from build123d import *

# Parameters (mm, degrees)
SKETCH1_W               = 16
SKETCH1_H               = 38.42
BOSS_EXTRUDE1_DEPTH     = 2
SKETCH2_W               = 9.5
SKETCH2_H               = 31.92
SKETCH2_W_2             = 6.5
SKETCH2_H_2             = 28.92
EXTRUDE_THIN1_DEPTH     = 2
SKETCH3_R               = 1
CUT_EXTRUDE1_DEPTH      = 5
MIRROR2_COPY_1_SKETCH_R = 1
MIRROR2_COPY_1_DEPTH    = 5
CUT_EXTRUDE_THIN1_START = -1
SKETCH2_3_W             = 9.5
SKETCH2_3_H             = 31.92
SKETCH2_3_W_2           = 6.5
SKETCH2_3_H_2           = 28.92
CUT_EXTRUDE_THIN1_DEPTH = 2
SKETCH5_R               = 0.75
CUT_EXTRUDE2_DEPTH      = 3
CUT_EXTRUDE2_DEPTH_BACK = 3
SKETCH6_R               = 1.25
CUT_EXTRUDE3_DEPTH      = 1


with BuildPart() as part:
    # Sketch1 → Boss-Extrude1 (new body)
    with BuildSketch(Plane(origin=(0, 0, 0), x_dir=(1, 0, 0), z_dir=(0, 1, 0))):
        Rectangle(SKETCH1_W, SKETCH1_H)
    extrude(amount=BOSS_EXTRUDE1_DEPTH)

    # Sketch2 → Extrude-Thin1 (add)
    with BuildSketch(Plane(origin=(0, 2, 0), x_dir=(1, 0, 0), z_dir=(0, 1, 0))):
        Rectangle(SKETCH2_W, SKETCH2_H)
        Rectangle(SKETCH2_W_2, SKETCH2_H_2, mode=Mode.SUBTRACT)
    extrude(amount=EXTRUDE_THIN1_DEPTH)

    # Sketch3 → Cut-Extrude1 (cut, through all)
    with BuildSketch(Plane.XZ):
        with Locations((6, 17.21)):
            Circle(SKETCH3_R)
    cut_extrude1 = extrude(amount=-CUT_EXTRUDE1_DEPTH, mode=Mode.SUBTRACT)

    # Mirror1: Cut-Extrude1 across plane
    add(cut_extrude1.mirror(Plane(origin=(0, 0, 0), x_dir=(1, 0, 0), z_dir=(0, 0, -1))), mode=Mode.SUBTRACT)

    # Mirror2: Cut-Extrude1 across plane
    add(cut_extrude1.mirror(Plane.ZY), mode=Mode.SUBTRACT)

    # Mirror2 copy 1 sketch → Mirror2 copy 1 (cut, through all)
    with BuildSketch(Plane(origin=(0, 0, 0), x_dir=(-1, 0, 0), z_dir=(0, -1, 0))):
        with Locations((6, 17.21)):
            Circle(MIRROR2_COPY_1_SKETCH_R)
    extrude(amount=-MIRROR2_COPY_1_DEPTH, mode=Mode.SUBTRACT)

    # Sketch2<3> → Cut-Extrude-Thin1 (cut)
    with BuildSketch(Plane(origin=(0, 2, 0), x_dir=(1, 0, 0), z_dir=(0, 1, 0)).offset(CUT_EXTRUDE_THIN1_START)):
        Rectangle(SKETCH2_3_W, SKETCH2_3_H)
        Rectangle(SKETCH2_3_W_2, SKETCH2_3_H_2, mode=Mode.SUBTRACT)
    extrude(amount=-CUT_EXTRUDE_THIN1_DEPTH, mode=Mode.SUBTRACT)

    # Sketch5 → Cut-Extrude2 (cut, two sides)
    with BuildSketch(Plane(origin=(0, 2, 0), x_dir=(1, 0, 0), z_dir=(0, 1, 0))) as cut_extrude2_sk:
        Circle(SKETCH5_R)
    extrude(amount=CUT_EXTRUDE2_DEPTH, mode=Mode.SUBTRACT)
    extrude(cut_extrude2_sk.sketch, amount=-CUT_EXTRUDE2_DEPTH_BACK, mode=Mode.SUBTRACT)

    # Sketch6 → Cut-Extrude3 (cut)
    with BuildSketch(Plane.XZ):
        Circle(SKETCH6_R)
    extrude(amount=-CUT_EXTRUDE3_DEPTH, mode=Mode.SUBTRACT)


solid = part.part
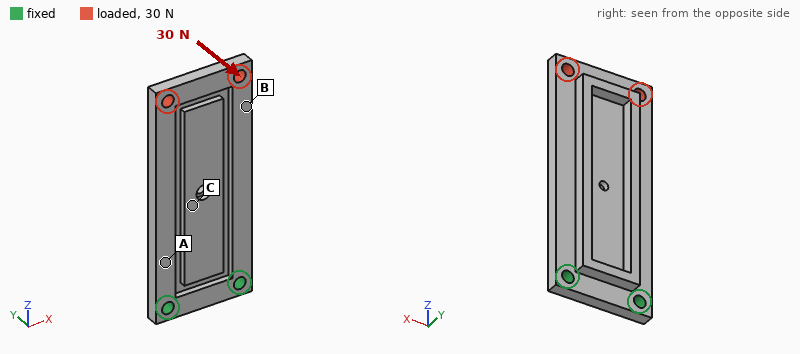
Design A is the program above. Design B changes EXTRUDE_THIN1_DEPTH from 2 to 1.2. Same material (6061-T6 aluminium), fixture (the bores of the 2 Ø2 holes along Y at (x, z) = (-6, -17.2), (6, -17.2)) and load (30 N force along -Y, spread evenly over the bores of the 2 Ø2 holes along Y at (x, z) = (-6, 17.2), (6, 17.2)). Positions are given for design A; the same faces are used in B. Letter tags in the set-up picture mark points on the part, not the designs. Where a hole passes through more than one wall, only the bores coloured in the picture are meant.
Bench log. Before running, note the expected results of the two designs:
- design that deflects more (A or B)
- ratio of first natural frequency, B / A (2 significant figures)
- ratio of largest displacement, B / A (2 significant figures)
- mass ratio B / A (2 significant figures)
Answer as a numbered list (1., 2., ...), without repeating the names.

1. B
2. 0.92
3. 1.3
4. 0.93
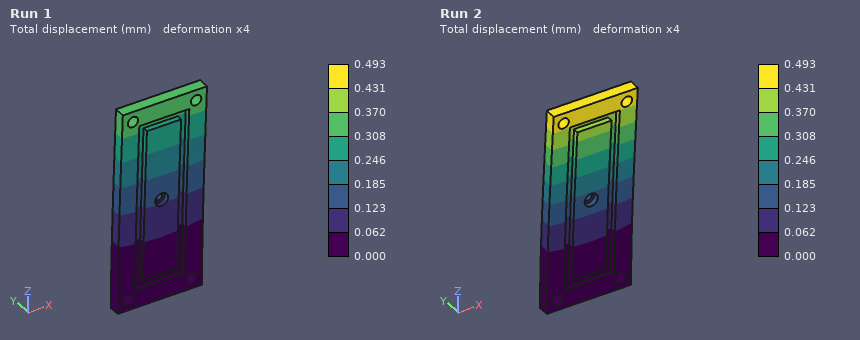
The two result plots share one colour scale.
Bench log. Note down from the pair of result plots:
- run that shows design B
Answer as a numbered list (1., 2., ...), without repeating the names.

1. Run 2
